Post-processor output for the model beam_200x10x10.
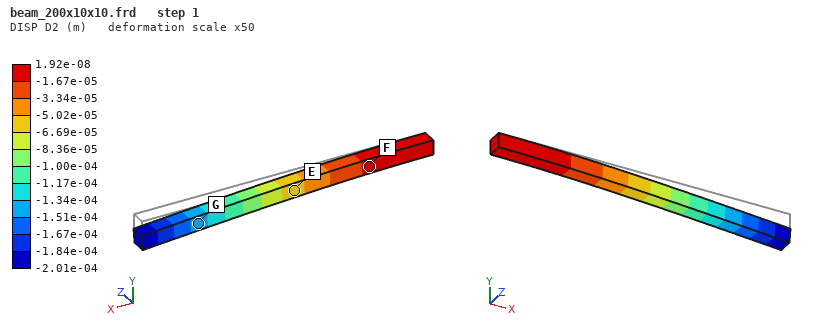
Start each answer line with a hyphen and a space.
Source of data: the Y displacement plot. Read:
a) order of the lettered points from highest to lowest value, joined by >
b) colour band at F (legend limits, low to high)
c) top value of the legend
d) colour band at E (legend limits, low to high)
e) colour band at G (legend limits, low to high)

- F > E > G
- -1.67e-05 to 1.92e-08 m
- 1.92e-08 m
- -6.69e-05 to -5.02e-05 m
- -1.51e-04 to -1.34e-04 m
